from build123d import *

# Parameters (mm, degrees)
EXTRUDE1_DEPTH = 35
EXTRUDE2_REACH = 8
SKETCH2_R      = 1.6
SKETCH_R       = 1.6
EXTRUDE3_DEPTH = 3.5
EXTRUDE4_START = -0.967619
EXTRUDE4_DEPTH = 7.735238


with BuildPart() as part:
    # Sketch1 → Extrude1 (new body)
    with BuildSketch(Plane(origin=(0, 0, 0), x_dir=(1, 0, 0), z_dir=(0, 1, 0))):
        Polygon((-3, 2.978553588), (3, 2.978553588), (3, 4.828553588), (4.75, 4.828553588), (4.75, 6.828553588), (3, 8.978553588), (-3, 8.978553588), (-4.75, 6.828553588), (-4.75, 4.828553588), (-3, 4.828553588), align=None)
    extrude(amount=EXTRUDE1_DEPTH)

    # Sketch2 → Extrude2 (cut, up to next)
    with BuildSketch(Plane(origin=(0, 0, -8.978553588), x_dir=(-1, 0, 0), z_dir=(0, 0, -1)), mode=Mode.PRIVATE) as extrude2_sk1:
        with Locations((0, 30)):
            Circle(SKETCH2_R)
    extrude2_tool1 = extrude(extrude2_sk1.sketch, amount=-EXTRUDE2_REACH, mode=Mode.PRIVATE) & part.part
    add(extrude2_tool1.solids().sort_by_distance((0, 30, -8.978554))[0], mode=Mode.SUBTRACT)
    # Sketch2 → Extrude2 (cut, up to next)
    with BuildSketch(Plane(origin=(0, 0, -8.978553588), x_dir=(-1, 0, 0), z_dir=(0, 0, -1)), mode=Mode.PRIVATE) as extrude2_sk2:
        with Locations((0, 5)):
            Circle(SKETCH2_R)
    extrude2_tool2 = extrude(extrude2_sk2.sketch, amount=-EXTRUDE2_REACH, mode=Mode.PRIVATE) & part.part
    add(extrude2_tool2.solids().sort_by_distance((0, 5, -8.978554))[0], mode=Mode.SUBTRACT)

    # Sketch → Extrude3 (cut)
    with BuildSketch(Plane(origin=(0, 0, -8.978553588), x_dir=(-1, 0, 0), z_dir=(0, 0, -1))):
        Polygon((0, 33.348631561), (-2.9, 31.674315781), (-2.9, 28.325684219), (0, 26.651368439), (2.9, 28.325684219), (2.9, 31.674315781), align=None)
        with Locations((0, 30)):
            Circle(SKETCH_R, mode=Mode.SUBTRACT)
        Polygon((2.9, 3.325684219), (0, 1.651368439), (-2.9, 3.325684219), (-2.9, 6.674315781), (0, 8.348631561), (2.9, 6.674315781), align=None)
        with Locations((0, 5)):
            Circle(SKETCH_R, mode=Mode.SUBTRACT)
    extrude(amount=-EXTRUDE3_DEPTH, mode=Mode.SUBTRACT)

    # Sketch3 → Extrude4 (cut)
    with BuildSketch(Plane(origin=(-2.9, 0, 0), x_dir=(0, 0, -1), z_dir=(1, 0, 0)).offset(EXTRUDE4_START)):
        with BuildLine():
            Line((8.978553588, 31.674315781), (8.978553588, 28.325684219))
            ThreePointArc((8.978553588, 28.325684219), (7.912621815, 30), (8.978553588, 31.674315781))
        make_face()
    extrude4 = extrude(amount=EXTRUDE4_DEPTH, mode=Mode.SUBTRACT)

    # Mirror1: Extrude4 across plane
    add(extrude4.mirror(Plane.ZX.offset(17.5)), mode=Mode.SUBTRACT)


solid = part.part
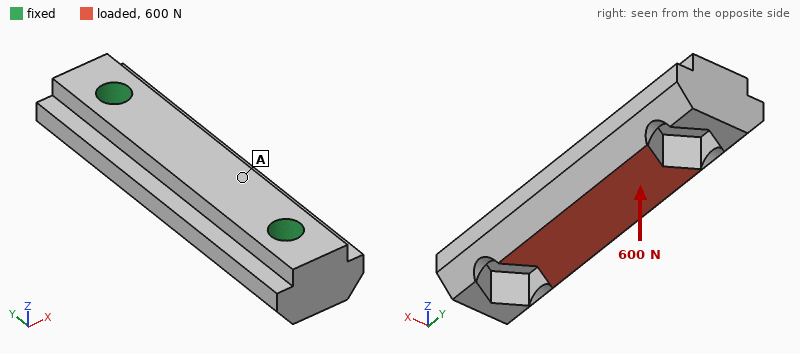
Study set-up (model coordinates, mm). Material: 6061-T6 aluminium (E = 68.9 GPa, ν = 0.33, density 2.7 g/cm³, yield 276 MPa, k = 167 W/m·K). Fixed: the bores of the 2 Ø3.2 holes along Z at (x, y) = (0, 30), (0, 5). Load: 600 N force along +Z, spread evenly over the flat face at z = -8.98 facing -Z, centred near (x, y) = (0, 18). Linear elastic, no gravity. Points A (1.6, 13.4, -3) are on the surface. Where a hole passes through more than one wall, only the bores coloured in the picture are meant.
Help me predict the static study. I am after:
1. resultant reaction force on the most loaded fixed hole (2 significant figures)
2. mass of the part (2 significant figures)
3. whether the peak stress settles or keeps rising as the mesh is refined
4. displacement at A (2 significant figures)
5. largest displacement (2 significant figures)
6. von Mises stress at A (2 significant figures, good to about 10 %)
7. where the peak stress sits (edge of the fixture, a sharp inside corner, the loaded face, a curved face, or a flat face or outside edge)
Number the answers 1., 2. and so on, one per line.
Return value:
1. 380 N
2. 3.7 g
3. keeps rising
4. 6.8 µm
5. 8.3 µm
6. 14 MPa
7. edge of the fixture
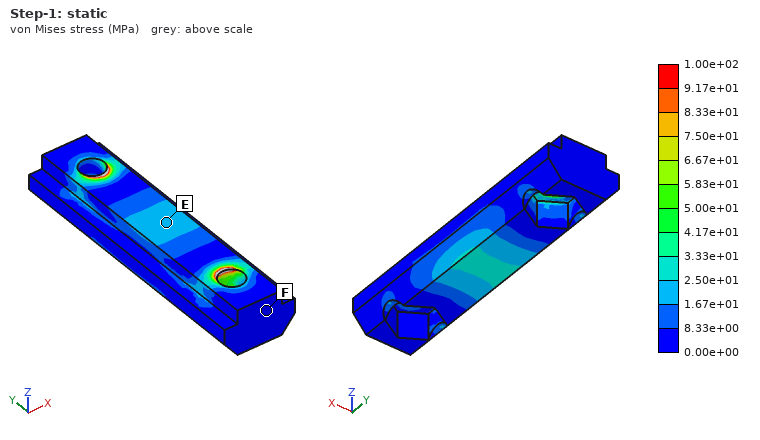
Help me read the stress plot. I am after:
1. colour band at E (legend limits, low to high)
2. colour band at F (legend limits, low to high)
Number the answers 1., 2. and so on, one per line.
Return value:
1. 1.67e+01 to 2.50e+01 MPa
2. 0.00e+00 to 8.33e+00 MPa
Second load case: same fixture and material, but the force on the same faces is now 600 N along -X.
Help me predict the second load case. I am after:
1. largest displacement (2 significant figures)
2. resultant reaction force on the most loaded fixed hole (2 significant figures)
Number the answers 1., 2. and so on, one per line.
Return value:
1. 20 µm
2. 300 N
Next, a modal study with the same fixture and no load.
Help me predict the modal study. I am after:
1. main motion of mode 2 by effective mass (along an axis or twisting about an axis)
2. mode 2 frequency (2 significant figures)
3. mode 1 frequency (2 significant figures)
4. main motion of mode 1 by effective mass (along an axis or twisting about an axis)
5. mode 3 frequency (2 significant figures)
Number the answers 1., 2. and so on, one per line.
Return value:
1. along Z
2. 30 kHz
3. 26 kHz
4. along X
5. 41 kHz
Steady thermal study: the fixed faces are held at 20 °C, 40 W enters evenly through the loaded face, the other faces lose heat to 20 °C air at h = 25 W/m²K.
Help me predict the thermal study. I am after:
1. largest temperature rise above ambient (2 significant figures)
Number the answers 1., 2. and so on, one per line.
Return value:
1. 31 K
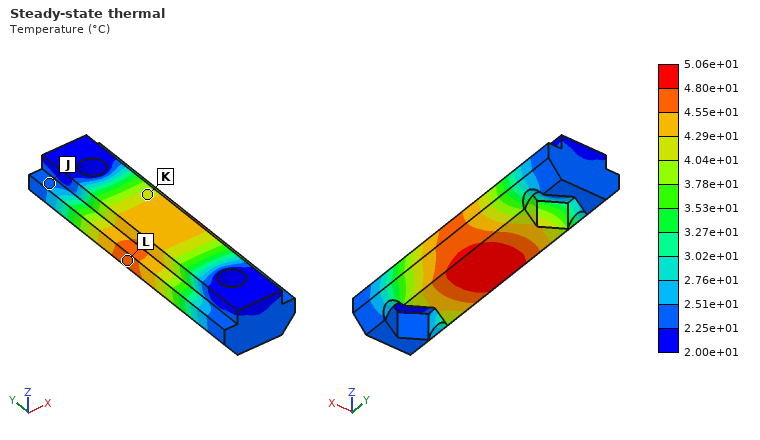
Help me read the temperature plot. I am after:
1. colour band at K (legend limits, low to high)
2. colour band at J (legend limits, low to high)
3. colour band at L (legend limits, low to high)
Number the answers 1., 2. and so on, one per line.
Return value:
1. 4.04e+01 to 4.29e+01 °C
2. 2.25e+01 to 2.51e+01 °C
3. 4.55e+01 to 4.80e+01 °C
